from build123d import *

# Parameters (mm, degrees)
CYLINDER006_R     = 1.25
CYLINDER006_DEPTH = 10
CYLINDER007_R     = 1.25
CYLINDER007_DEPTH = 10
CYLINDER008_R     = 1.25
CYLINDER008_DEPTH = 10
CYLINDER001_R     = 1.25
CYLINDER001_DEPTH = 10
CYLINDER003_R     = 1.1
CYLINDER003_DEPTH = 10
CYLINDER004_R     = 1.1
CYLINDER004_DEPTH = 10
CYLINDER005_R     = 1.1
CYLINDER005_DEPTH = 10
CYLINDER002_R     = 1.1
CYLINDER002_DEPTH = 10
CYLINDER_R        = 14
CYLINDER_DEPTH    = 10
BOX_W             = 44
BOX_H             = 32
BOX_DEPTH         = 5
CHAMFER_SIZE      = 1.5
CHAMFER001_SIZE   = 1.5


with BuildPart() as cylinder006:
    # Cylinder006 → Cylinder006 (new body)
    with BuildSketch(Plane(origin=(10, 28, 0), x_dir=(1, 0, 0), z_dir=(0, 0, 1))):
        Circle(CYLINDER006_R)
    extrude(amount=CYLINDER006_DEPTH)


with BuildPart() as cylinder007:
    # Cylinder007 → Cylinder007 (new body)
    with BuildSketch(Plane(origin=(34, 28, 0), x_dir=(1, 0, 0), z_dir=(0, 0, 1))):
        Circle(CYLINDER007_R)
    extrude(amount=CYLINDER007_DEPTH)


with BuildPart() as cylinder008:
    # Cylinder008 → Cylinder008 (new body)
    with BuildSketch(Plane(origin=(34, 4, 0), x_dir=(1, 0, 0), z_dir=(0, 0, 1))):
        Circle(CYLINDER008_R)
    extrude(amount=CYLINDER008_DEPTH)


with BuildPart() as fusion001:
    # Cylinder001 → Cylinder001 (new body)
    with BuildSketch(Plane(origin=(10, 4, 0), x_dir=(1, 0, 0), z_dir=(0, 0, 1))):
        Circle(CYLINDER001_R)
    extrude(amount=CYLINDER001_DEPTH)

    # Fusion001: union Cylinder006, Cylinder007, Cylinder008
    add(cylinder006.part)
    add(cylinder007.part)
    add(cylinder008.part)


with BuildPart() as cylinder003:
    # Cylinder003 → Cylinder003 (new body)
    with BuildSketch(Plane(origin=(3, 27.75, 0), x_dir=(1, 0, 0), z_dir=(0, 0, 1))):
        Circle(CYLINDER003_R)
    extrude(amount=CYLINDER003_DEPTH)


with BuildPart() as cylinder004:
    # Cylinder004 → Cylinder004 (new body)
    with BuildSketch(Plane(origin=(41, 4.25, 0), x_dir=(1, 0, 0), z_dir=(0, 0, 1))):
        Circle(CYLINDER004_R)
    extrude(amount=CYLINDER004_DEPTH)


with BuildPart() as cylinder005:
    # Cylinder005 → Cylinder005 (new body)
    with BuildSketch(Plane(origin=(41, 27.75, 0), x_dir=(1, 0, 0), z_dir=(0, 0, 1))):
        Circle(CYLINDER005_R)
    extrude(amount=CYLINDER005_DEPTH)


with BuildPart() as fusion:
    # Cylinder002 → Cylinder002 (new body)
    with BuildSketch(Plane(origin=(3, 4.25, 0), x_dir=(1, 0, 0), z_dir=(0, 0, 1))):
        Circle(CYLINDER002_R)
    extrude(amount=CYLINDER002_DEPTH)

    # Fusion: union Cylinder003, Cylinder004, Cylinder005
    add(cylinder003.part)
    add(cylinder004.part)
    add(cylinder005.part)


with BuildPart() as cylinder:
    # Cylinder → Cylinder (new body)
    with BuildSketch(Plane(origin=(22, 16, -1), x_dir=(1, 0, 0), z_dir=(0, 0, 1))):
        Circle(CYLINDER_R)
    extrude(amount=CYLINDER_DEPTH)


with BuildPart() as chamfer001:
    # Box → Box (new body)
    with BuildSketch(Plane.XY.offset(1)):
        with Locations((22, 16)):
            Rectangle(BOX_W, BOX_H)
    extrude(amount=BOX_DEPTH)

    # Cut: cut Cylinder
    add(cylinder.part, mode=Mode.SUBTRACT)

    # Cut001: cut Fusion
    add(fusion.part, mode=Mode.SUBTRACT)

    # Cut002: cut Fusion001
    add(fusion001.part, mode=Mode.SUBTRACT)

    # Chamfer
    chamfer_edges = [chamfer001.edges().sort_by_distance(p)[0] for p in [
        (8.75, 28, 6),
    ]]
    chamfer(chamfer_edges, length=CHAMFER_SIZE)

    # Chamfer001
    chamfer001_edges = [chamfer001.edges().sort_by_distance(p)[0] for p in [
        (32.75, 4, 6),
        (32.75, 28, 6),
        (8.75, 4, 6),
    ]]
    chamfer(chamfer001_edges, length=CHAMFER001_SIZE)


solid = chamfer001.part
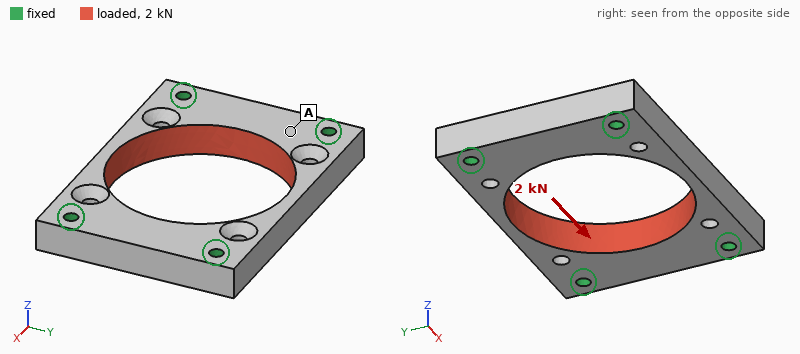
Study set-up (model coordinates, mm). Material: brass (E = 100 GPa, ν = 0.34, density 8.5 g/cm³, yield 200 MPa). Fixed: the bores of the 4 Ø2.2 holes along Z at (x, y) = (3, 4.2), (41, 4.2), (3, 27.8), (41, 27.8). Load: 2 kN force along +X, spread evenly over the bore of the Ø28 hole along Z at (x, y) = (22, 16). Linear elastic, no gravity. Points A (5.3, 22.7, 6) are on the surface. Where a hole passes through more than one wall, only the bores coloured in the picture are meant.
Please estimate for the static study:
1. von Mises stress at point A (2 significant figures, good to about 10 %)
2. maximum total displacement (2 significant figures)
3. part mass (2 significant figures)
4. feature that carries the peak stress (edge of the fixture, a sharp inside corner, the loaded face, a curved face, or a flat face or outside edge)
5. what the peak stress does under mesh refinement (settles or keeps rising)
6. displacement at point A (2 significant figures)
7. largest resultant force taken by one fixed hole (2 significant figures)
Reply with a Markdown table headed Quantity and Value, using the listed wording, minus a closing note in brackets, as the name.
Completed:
| Quantity | Value |
|---|---|
| von Mises stress at point A | 8.9 MPa |
| maximum total displacement | 2.4 µm |
| part mass | 32 g |
| feature that carries the peak stress | edge of the fixture |
| what the peak stress does under mesh refinement | keeps rising |
| displacement at point A | 1.3 µm |
| largest resultant force taken by one fixed hole | 510 N |
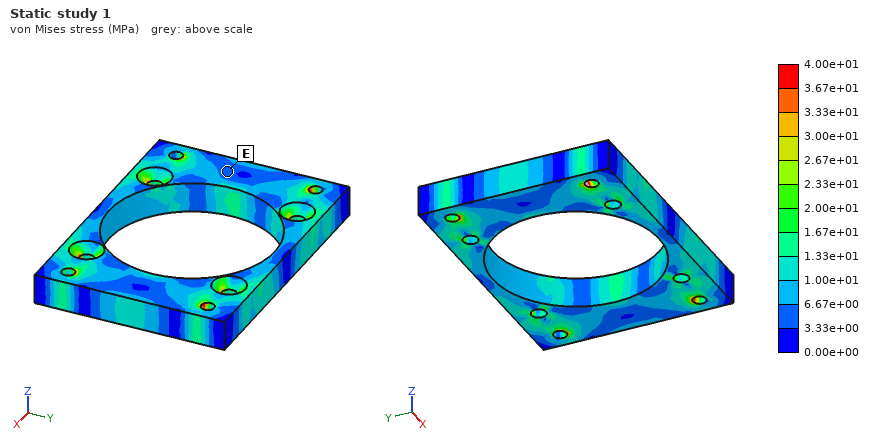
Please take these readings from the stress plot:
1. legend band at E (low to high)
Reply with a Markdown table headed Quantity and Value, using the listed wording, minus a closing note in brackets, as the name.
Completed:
| Quantity | Value |
|---|---|
| legend band at E | 3.33e+00 to 6.67e+00 MPa |
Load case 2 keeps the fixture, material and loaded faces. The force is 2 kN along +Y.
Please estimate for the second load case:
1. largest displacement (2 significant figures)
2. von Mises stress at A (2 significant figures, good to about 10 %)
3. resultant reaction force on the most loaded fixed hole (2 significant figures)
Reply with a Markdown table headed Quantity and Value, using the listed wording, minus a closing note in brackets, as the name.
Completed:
| Quantity | Value |
|---|---|
| largest displacement | 15 µm |
| von Mises stress at A | 15 MPa |
| resultant reaction force on the most loaded fixed hole | 500 N |
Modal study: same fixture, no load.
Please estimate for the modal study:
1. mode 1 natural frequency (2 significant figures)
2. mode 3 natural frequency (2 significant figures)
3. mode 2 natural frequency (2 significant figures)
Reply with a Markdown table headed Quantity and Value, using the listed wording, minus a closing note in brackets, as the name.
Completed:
| Quantity | Value |
|---|---|
| mode 1 natural frequency | 14 kHz |
| mode 3 natural frequency | 18 kHz |
| mode 2 natural frequency | 14 kHz |
